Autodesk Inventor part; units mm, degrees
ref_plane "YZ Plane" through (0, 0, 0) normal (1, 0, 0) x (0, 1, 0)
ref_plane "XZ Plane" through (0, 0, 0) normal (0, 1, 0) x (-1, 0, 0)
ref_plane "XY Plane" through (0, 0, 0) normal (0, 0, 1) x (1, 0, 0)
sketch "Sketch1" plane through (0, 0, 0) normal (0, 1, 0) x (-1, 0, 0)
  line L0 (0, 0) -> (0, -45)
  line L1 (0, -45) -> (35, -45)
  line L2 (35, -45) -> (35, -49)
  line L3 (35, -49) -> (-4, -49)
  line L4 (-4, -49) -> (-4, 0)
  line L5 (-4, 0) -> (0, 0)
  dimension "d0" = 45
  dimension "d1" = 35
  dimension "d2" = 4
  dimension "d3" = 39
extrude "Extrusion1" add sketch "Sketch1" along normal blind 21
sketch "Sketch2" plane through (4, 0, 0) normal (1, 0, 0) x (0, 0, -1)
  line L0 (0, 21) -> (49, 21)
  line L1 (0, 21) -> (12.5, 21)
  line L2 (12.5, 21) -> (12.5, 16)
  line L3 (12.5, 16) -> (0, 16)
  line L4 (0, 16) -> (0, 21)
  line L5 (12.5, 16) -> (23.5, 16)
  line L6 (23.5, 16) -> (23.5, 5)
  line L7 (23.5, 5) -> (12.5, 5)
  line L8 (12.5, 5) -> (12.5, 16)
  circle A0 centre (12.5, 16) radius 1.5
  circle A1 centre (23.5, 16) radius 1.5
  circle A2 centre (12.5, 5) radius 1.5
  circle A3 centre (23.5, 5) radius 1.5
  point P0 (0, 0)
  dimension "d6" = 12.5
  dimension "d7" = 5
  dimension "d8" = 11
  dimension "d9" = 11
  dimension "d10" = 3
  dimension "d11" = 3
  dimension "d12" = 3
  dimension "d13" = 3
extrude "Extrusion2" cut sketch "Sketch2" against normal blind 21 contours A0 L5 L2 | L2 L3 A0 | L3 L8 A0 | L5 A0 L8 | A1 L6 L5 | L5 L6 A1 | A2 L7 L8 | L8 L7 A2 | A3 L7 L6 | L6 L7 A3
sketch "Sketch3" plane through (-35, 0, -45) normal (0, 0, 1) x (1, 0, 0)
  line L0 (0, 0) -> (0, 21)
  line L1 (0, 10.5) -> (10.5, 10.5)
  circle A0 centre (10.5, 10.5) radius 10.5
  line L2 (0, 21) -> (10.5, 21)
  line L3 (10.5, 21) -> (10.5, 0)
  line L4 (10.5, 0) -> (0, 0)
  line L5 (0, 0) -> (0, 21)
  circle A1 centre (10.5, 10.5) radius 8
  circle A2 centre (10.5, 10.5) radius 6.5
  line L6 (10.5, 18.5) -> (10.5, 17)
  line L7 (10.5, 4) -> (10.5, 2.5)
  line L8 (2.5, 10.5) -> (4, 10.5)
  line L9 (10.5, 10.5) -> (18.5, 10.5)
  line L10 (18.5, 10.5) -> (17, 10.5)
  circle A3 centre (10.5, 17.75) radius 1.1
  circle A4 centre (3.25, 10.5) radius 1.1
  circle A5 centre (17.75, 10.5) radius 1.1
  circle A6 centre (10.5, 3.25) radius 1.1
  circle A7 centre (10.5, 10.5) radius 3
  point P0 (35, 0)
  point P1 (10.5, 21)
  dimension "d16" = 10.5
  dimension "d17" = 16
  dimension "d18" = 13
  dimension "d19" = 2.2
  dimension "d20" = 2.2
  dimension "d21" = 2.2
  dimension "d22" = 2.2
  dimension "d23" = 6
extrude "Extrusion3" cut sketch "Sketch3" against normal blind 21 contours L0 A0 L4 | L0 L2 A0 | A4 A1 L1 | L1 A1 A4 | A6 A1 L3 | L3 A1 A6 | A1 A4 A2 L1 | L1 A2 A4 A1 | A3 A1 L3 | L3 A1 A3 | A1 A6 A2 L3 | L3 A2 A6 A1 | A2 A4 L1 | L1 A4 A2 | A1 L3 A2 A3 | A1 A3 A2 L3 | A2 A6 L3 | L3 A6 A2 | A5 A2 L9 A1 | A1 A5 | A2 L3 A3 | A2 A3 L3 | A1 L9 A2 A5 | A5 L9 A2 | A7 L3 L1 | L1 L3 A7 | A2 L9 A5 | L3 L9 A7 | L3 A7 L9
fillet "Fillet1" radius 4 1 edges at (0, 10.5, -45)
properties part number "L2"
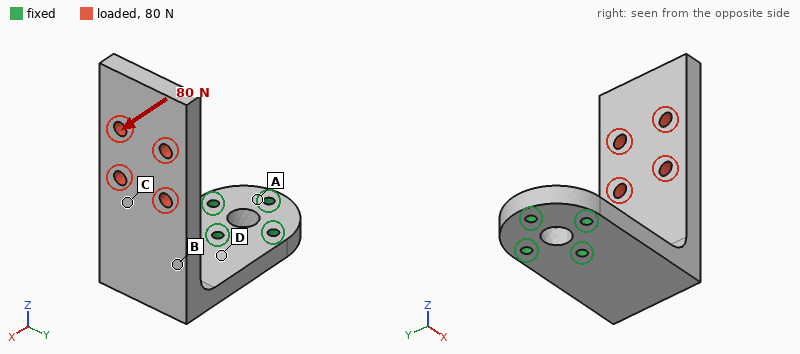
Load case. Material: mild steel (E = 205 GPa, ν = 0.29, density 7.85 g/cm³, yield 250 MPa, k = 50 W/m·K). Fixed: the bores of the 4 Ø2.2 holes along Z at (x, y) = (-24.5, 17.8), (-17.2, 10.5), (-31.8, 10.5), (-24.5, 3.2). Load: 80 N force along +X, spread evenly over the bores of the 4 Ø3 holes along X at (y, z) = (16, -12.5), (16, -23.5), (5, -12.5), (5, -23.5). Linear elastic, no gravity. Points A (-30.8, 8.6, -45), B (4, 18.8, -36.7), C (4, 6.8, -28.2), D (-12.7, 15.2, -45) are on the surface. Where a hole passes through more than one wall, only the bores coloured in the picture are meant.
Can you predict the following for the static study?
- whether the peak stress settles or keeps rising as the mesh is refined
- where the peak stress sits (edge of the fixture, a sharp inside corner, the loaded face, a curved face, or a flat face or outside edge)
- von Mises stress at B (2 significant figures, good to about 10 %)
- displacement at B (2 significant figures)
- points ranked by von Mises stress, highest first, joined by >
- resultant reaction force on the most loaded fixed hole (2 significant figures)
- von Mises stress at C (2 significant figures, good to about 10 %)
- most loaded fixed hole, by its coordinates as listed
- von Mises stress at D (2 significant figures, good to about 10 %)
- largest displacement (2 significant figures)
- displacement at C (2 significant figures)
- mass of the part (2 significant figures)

keeps rising
edge of the fixture
27 MPa
0.032 mm
D > B > C > A
170 N
14 MPa
(-17.2, 10.5)
39 MPa
0.13 mm
0.049 mm
52 g
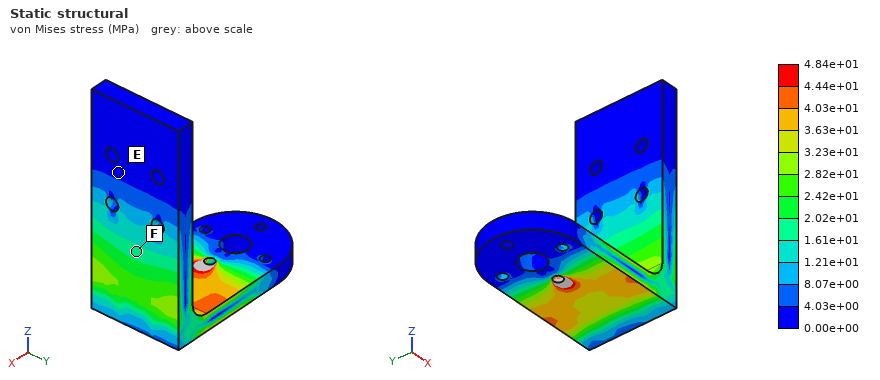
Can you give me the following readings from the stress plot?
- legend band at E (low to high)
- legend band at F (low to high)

0.00e+00 to 4.03e+00 MPa
1.61e+01 to 2.02e+01 MPa
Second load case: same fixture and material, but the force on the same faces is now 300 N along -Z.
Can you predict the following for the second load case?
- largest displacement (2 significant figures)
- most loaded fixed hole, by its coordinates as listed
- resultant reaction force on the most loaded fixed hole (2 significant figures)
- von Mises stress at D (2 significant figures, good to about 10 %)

0.13 mm
(-17.2, 10.5)
620 N
71 MPa
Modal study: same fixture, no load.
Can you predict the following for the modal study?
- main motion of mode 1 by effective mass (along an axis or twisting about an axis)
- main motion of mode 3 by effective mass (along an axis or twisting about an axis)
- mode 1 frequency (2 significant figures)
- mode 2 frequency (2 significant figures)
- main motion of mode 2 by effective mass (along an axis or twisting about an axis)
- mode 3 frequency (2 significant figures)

along X
along Z
960 Hz
1500 Hz
along Y
3500 Hz
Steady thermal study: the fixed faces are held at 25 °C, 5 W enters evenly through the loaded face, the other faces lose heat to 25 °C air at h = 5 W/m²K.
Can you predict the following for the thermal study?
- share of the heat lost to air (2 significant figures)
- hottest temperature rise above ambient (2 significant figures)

11 %
53 K
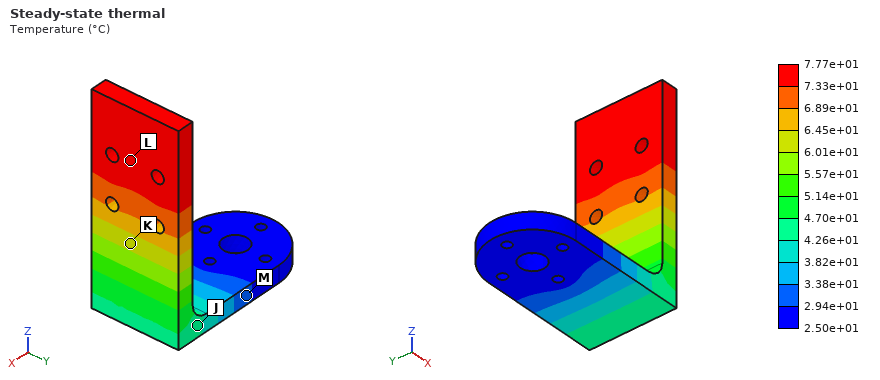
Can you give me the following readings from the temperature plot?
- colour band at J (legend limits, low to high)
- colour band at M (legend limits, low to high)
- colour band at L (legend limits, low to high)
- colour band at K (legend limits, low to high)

4.26e+01 to 4.70e+01 °C
2.94e+01 to 3.38e+01 °C
7.33e+01 to 7.77e+01 °C
6.01e+01 to 6.45e+01 °C
